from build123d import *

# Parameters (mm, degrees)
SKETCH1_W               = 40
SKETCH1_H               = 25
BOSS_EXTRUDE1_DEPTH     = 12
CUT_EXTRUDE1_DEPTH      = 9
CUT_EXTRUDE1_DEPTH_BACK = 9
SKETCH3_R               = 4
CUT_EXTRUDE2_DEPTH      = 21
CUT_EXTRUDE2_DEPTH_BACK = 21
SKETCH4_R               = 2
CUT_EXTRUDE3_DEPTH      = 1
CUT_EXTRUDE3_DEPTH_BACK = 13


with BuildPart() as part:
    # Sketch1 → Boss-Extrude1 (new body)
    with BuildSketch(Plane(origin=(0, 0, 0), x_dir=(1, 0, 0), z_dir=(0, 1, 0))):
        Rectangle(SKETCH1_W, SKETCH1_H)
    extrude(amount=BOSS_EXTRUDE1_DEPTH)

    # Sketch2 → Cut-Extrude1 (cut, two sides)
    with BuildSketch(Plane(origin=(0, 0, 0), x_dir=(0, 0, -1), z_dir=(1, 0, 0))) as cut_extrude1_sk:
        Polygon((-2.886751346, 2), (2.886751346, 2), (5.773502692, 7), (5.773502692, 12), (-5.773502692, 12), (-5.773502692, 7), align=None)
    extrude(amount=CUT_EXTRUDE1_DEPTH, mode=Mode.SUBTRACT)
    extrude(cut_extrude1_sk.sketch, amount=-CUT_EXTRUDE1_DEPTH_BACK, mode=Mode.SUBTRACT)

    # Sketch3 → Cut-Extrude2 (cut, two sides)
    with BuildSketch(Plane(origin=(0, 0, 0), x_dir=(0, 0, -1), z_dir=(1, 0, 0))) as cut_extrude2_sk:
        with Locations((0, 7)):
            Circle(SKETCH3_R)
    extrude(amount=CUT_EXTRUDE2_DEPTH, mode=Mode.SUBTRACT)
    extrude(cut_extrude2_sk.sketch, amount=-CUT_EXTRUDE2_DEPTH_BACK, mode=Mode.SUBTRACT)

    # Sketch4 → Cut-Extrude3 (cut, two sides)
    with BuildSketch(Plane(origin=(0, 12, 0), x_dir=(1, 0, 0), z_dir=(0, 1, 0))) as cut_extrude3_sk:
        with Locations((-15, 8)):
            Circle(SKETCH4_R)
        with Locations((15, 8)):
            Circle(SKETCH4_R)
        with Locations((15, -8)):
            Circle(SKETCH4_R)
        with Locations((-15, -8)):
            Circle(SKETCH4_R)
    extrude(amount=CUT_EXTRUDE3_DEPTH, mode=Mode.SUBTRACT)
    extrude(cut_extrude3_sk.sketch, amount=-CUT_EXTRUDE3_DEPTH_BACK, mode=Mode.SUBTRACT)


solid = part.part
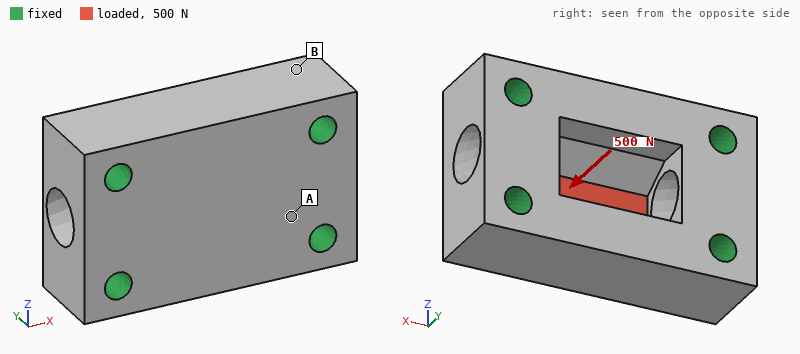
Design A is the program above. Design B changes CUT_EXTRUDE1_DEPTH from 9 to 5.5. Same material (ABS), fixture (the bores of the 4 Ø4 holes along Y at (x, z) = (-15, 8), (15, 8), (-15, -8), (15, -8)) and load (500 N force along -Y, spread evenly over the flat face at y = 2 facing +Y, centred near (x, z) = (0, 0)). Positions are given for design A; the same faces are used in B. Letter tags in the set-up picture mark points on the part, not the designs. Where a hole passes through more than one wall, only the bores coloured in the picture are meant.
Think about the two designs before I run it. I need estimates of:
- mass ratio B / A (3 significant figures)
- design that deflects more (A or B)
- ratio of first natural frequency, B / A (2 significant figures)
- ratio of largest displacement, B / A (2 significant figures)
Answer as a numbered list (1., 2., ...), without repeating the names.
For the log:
1. 1.02
2. B
3. 1.0
4. 1.1
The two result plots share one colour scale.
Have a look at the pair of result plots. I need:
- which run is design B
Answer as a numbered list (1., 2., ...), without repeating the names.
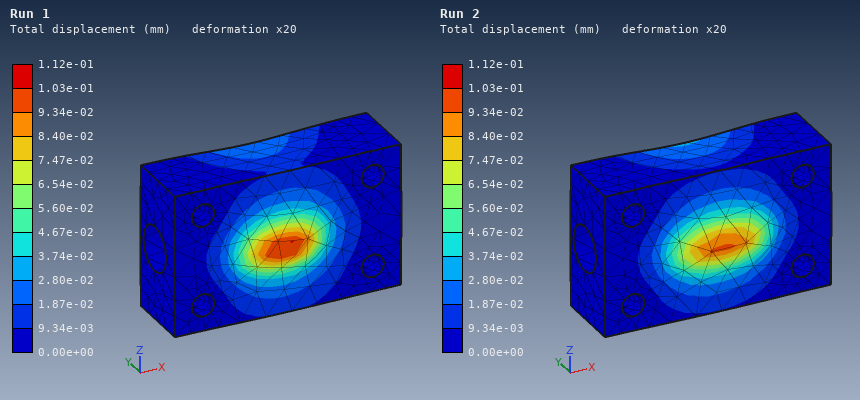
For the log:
1. Run 1
